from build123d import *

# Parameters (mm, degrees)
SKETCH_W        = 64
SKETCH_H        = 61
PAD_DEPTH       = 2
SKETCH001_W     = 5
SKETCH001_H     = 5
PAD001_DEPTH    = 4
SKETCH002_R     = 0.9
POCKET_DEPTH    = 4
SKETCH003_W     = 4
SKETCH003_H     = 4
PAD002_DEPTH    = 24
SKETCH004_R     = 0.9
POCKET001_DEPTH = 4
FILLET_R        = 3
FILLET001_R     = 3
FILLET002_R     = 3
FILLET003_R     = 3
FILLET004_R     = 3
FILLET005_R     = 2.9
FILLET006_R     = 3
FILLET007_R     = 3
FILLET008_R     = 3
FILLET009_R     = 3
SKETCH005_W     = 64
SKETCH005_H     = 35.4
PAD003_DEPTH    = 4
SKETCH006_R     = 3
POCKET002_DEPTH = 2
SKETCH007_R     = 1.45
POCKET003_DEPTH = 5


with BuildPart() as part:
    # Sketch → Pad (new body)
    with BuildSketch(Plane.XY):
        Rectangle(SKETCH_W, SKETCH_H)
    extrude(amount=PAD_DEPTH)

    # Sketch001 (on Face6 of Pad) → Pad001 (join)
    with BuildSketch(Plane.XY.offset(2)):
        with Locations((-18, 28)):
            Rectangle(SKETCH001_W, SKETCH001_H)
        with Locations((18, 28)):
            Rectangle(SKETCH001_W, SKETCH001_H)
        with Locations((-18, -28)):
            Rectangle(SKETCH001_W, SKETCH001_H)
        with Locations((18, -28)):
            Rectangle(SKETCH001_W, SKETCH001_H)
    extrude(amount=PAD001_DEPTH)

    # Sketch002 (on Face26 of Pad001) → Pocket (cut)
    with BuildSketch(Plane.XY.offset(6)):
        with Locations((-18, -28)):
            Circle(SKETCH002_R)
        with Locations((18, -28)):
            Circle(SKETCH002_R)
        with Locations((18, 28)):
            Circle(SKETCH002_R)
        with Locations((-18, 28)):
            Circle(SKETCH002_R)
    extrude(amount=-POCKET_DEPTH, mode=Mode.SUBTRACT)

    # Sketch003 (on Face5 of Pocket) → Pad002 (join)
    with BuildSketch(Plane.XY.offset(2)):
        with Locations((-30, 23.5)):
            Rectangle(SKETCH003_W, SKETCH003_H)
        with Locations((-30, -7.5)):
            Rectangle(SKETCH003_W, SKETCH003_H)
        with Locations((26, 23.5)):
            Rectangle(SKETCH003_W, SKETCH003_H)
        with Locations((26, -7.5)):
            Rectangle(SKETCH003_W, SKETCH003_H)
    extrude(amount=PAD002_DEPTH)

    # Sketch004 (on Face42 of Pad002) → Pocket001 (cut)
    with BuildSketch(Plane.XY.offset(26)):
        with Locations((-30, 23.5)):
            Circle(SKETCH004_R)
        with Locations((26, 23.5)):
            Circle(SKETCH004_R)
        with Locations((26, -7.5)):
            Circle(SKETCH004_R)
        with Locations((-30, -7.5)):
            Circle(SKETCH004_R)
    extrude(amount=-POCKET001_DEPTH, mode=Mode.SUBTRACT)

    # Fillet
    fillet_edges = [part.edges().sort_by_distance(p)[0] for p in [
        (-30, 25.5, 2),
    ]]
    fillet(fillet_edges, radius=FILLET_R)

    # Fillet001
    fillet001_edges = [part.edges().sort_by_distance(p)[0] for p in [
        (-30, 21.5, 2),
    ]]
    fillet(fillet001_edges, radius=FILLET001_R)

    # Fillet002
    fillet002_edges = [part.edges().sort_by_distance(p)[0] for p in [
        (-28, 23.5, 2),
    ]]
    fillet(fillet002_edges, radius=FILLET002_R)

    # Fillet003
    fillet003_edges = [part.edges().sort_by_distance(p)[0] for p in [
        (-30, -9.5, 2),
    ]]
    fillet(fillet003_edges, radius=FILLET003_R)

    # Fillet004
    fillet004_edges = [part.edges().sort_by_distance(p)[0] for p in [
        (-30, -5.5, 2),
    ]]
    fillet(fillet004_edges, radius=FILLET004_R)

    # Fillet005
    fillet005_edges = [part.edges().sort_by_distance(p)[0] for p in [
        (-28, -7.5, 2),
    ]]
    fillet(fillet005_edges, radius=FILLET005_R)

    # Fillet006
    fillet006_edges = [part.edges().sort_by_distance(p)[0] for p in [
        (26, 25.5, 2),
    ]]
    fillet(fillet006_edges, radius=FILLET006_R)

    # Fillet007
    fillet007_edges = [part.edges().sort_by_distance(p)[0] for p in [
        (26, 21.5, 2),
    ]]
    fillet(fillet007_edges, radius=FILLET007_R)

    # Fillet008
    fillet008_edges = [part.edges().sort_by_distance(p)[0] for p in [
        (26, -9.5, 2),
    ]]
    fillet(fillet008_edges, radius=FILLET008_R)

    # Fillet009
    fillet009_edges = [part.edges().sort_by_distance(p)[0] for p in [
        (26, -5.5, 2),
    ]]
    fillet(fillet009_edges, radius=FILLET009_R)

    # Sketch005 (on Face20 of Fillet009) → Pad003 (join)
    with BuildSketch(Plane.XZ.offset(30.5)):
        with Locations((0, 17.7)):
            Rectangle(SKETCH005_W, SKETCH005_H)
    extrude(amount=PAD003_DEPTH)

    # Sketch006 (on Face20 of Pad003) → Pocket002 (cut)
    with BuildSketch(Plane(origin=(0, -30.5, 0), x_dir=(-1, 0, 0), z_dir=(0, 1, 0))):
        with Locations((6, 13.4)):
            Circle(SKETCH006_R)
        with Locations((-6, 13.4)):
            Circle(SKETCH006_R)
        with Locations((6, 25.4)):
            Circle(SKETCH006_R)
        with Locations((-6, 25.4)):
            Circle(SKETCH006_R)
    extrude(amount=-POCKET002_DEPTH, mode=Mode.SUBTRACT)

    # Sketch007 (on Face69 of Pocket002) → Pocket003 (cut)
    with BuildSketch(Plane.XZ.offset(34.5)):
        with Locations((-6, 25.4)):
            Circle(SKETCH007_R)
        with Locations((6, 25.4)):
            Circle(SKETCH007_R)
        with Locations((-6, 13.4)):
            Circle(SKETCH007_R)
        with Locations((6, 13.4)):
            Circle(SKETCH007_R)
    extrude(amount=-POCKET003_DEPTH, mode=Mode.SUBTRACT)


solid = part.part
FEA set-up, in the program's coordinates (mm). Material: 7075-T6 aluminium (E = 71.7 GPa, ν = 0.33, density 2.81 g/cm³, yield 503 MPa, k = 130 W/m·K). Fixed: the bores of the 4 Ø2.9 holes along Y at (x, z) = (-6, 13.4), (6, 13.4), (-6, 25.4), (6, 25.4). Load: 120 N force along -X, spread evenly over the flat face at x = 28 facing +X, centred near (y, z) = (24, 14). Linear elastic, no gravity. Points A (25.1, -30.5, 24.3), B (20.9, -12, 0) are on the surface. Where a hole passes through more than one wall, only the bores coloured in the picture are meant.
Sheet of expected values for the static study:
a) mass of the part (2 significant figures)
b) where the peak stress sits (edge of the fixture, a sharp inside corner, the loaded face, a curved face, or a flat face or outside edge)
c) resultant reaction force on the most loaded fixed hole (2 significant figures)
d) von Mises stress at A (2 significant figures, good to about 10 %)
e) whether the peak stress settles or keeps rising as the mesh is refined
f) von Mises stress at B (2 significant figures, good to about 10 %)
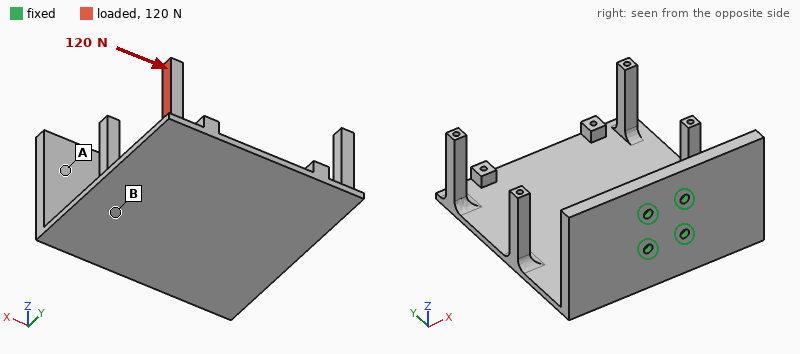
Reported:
52 g
edge of the fixture
490 N
13 MPa
keeps rising
36 MPa
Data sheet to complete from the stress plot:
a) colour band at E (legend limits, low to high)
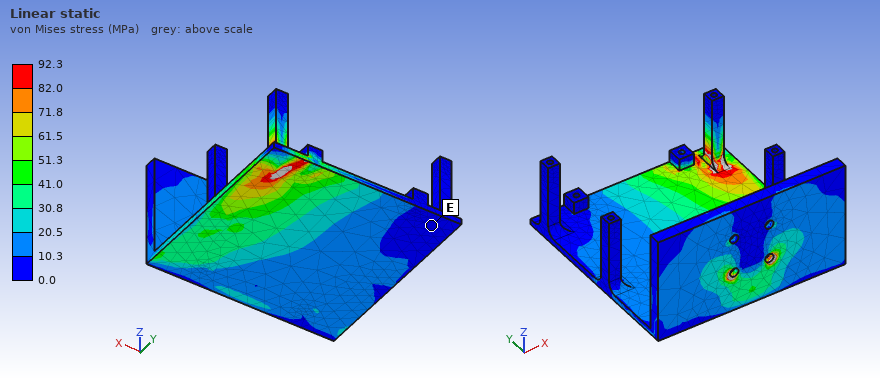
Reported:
0.0 to 10.3 MPa
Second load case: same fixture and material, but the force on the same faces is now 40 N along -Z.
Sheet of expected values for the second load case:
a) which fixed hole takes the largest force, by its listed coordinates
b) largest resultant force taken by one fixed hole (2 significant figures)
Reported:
(6, 25.4)
140 N
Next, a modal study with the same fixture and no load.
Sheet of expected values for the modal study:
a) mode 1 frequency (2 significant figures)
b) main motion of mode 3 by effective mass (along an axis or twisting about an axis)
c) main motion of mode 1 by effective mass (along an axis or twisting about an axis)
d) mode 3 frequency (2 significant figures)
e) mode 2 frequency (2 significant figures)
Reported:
380 Hz
along X
along Z
1100 Hz
740 Hz
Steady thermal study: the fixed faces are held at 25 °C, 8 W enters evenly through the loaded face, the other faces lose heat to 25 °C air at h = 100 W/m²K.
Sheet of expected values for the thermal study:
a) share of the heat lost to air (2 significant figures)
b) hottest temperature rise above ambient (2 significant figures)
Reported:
83 %
57 K
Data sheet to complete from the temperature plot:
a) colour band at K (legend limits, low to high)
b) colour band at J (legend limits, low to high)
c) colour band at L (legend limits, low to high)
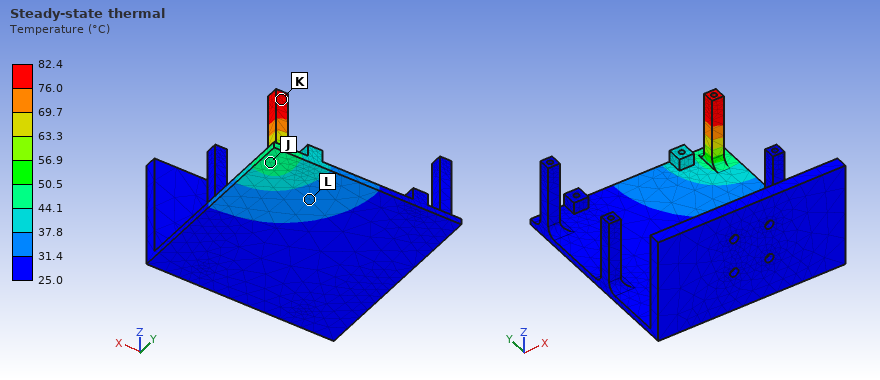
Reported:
76.0 to 82.4 °C
44.1 to 50.5 °C
31.4 to 37.8 °C
